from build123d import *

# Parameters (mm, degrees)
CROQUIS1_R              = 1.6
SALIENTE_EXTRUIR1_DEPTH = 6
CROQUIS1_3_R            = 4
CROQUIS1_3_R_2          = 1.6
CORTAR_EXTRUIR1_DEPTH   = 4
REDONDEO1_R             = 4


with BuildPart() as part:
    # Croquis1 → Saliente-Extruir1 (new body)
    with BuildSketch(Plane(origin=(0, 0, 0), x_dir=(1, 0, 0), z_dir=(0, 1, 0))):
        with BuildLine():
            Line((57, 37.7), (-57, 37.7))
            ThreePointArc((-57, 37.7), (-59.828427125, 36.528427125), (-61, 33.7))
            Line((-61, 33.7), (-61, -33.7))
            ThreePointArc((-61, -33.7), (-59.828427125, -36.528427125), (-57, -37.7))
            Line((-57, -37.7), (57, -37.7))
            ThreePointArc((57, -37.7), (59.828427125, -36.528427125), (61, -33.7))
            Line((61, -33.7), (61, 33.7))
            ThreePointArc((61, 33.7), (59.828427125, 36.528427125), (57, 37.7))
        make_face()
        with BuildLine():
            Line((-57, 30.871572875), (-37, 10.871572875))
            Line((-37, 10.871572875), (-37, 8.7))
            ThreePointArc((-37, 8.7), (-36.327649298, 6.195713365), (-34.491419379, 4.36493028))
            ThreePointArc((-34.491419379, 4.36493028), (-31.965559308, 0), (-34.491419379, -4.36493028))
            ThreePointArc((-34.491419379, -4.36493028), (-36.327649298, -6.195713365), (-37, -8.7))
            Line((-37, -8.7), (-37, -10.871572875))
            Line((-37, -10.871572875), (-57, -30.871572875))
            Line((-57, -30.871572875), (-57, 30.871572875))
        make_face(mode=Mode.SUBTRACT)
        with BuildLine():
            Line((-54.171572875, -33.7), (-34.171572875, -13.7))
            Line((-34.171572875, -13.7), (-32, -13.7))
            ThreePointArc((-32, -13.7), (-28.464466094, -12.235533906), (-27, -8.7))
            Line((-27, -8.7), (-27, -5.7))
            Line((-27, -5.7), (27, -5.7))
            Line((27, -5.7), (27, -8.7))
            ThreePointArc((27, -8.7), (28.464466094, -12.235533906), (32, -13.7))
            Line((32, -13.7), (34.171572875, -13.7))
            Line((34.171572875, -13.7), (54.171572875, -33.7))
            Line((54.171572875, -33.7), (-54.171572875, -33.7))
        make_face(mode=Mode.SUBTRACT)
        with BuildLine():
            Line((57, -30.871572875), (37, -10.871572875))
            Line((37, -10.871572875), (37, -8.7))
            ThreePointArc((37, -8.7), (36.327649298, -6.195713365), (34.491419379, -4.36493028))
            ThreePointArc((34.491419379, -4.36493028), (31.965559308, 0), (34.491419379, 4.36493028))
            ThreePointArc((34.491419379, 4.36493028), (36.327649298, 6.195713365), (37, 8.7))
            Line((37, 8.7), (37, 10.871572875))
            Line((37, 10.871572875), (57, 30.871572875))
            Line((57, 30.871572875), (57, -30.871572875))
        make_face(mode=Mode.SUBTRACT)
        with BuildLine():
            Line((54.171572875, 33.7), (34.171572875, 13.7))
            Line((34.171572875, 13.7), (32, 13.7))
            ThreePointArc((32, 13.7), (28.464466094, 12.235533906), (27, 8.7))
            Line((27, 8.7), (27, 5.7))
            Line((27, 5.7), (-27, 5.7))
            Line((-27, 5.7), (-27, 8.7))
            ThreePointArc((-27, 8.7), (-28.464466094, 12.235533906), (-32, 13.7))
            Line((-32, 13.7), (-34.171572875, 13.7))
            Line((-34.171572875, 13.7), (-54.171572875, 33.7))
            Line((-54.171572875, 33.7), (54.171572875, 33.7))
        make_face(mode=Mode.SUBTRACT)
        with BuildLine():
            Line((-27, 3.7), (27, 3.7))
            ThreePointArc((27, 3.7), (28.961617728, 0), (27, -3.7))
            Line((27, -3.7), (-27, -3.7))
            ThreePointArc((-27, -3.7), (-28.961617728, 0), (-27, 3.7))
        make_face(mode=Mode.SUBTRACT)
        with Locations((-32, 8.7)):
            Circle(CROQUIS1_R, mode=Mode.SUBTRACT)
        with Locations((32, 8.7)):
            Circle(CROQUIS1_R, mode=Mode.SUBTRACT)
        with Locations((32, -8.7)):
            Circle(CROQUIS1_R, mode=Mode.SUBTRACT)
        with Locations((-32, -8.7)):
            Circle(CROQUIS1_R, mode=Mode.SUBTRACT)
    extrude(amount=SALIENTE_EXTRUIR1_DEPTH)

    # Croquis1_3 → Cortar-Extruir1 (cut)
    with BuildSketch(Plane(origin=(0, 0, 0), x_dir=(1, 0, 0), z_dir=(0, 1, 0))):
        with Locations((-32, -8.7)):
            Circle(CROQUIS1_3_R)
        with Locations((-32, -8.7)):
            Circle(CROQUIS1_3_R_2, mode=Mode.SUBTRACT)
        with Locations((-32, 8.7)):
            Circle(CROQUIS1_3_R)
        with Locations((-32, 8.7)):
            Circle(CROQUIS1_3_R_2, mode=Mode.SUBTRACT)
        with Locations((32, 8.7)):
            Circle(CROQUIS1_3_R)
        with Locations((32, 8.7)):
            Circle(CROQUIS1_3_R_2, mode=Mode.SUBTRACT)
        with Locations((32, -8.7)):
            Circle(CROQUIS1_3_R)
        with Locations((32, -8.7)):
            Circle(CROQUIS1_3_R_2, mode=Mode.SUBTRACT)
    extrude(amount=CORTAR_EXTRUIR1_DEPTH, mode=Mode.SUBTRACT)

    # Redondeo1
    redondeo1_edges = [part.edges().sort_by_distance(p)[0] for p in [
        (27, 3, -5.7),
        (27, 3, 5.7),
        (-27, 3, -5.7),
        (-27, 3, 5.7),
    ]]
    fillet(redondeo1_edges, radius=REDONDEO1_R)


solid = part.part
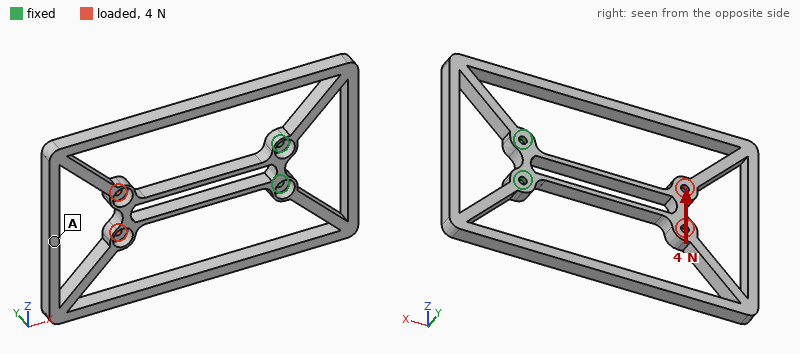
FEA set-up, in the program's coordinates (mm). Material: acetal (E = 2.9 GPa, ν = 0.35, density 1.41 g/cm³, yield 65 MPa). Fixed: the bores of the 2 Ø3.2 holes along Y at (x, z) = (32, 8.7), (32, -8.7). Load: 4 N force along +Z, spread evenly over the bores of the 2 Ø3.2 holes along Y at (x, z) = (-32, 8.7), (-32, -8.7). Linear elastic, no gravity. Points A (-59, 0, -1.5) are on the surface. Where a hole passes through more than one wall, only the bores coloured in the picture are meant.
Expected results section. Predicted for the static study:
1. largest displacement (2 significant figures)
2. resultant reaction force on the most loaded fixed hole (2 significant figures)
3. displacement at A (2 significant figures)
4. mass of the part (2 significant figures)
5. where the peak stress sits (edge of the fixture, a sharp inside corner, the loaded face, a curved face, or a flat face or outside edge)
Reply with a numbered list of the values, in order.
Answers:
1. 1.5 mm
2. 12 N
3. 1.5 mm
4. 21 g
5. a curved face
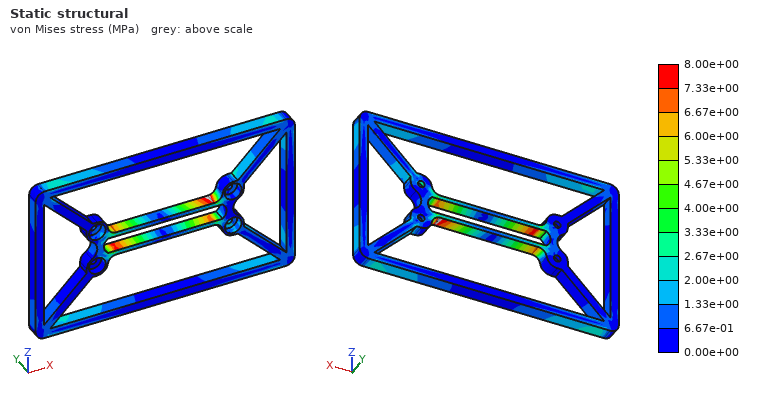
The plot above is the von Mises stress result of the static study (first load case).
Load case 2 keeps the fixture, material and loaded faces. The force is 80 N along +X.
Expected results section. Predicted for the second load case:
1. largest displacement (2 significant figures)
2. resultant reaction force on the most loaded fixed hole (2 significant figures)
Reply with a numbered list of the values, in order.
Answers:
1. 1.6 mm
2. 45 N
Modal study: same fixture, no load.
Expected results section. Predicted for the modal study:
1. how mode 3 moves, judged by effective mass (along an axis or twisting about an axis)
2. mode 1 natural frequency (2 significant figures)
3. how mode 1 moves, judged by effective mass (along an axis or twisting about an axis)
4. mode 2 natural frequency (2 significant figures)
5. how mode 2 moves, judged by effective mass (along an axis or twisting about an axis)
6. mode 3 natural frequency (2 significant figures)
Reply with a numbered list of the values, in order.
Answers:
1. twisting about X
2. 70 Hz
3. along Y
4. 85 Hz
5. along Z
6. 130 Hz
